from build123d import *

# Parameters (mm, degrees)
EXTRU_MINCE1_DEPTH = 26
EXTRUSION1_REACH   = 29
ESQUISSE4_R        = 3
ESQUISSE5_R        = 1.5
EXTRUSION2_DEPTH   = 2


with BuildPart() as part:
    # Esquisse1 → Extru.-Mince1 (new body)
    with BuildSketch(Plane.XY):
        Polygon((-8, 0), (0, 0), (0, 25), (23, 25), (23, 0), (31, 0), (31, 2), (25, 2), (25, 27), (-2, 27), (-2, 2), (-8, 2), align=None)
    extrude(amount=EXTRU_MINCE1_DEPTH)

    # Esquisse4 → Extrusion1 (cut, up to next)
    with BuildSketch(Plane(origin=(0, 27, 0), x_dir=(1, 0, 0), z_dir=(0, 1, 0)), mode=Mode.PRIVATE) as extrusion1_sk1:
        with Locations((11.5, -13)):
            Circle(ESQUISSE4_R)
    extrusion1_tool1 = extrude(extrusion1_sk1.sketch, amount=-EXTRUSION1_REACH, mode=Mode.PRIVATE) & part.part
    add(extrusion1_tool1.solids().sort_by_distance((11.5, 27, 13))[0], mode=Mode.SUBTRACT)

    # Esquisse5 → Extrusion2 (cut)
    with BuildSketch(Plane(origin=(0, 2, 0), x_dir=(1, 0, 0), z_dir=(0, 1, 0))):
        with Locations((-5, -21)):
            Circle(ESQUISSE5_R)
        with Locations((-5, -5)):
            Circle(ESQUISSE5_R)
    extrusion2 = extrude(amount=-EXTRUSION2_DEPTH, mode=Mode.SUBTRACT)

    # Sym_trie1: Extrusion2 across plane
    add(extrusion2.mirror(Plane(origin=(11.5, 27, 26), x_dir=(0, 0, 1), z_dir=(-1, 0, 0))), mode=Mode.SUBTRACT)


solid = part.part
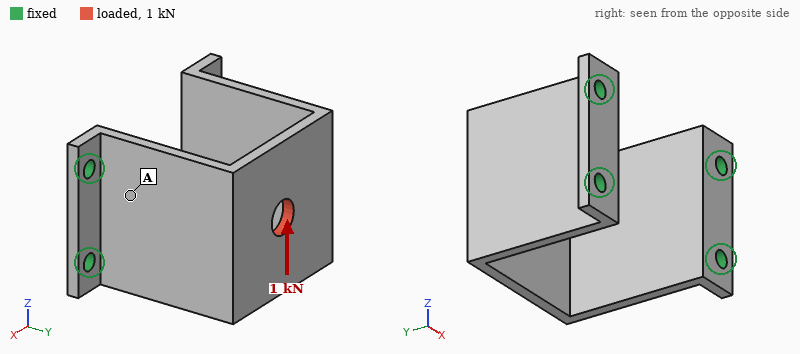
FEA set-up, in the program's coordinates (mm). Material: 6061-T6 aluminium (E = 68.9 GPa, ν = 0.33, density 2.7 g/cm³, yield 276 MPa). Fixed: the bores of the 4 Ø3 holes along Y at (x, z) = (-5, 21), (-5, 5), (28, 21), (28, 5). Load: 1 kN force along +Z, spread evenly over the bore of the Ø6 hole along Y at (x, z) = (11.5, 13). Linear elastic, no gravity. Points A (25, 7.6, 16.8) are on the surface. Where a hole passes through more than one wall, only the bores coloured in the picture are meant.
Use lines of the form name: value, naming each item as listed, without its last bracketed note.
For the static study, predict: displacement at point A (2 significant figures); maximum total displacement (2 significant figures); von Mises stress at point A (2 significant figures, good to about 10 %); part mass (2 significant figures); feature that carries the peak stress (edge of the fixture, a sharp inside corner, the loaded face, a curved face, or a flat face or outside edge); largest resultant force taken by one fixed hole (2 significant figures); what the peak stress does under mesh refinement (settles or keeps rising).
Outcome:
displacement at point A: 24 µm
maximum total displacement: 90 µm
von Mises stress at point A: 41 MPa
part mass: 12 g
feature that carries the peak stress: edge of the fixture
largest resultant force taken by one fixed hole: 770 N
what the peak stress does under mesh refinement: keeps rising
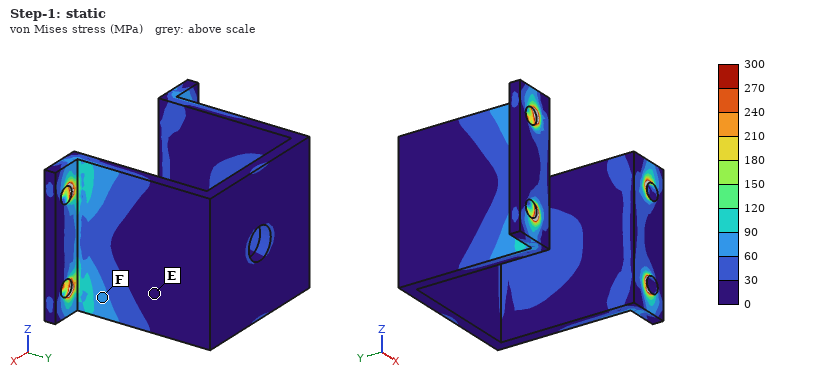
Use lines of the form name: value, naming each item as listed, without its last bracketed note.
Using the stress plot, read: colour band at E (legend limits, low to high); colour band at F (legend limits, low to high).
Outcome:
colour band at E: 0 to 30 MPa
colour band at F: 60 to 90 MPa
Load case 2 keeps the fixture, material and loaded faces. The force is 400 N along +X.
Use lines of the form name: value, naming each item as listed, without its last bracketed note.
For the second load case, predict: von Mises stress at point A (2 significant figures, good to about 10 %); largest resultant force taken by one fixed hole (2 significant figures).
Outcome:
von Mises stress at point A: 66 MPa
largest resultant force taken by one fixed hole: 140 N
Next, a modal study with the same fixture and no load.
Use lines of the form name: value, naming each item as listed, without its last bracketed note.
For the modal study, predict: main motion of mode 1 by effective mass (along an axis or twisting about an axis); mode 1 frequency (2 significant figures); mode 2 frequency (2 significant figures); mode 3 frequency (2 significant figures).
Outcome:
main motion of mode 1 by effective mass: along X
mode 1 frequency: 2200 Hz
mode 2 frequency: 6800 Hz
mode 3 frequency: 7100 Hz
